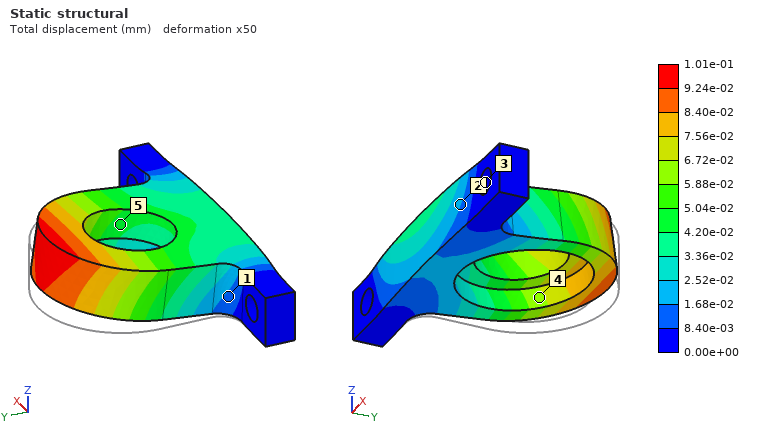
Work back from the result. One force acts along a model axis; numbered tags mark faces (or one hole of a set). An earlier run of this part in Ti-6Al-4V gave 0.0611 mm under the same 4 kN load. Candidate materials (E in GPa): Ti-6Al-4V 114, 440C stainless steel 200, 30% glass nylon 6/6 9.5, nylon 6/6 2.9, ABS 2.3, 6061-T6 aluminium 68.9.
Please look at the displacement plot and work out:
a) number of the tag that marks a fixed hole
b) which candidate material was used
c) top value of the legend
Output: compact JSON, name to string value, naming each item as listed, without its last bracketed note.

{"number of the tag that marks a fixed hole": "3", "which candidate material was used": "6061-T6 aluminium", "top value of the legend": "1.01e-01 mm"}
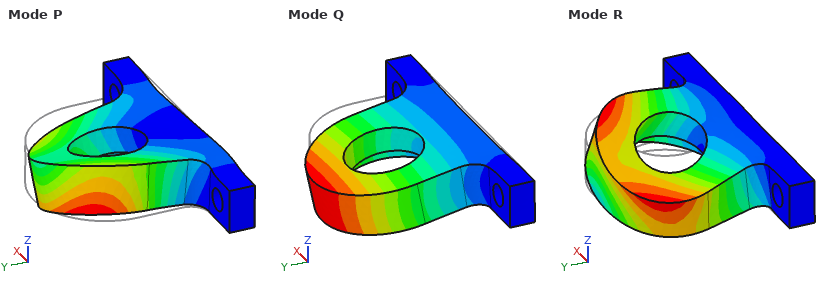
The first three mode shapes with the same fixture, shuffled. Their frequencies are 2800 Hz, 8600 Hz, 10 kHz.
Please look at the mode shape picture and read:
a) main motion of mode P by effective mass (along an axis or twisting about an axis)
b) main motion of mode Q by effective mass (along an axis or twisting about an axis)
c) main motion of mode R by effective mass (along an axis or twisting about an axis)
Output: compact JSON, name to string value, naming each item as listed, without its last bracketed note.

{"main motion of mode P by effective mass": "along X", "main motion of mode Q by effective mass": "along Z", "main motion of mode R by effective mass": "along X"}
